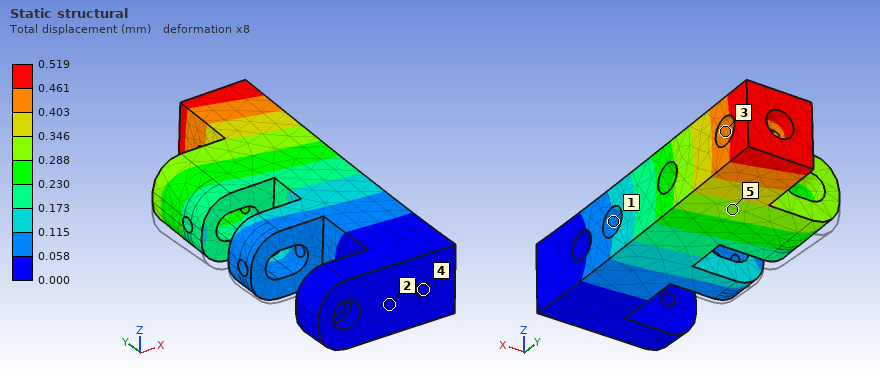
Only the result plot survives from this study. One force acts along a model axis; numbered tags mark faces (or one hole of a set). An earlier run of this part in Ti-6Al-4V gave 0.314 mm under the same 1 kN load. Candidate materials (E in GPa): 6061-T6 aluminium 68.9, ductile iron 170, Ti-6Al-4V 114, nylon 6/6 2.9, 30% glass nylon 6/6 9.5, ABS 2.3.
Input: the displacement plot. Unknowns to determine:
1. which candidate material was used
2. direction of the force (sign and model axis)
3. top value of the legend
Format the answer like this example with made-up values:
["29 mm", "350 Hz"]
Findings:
["6061-T6 aluminium", "+Z", "0.519 mm"]
